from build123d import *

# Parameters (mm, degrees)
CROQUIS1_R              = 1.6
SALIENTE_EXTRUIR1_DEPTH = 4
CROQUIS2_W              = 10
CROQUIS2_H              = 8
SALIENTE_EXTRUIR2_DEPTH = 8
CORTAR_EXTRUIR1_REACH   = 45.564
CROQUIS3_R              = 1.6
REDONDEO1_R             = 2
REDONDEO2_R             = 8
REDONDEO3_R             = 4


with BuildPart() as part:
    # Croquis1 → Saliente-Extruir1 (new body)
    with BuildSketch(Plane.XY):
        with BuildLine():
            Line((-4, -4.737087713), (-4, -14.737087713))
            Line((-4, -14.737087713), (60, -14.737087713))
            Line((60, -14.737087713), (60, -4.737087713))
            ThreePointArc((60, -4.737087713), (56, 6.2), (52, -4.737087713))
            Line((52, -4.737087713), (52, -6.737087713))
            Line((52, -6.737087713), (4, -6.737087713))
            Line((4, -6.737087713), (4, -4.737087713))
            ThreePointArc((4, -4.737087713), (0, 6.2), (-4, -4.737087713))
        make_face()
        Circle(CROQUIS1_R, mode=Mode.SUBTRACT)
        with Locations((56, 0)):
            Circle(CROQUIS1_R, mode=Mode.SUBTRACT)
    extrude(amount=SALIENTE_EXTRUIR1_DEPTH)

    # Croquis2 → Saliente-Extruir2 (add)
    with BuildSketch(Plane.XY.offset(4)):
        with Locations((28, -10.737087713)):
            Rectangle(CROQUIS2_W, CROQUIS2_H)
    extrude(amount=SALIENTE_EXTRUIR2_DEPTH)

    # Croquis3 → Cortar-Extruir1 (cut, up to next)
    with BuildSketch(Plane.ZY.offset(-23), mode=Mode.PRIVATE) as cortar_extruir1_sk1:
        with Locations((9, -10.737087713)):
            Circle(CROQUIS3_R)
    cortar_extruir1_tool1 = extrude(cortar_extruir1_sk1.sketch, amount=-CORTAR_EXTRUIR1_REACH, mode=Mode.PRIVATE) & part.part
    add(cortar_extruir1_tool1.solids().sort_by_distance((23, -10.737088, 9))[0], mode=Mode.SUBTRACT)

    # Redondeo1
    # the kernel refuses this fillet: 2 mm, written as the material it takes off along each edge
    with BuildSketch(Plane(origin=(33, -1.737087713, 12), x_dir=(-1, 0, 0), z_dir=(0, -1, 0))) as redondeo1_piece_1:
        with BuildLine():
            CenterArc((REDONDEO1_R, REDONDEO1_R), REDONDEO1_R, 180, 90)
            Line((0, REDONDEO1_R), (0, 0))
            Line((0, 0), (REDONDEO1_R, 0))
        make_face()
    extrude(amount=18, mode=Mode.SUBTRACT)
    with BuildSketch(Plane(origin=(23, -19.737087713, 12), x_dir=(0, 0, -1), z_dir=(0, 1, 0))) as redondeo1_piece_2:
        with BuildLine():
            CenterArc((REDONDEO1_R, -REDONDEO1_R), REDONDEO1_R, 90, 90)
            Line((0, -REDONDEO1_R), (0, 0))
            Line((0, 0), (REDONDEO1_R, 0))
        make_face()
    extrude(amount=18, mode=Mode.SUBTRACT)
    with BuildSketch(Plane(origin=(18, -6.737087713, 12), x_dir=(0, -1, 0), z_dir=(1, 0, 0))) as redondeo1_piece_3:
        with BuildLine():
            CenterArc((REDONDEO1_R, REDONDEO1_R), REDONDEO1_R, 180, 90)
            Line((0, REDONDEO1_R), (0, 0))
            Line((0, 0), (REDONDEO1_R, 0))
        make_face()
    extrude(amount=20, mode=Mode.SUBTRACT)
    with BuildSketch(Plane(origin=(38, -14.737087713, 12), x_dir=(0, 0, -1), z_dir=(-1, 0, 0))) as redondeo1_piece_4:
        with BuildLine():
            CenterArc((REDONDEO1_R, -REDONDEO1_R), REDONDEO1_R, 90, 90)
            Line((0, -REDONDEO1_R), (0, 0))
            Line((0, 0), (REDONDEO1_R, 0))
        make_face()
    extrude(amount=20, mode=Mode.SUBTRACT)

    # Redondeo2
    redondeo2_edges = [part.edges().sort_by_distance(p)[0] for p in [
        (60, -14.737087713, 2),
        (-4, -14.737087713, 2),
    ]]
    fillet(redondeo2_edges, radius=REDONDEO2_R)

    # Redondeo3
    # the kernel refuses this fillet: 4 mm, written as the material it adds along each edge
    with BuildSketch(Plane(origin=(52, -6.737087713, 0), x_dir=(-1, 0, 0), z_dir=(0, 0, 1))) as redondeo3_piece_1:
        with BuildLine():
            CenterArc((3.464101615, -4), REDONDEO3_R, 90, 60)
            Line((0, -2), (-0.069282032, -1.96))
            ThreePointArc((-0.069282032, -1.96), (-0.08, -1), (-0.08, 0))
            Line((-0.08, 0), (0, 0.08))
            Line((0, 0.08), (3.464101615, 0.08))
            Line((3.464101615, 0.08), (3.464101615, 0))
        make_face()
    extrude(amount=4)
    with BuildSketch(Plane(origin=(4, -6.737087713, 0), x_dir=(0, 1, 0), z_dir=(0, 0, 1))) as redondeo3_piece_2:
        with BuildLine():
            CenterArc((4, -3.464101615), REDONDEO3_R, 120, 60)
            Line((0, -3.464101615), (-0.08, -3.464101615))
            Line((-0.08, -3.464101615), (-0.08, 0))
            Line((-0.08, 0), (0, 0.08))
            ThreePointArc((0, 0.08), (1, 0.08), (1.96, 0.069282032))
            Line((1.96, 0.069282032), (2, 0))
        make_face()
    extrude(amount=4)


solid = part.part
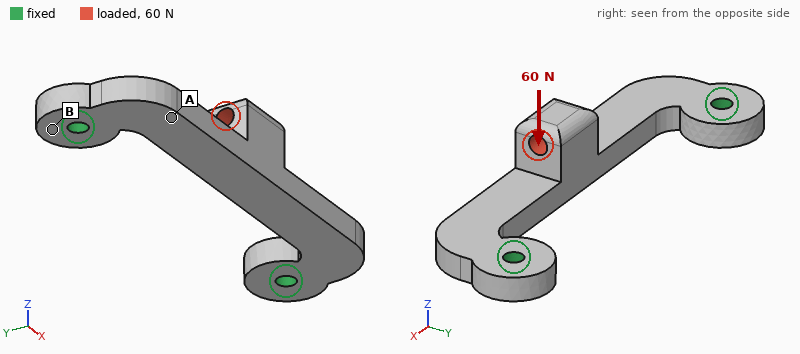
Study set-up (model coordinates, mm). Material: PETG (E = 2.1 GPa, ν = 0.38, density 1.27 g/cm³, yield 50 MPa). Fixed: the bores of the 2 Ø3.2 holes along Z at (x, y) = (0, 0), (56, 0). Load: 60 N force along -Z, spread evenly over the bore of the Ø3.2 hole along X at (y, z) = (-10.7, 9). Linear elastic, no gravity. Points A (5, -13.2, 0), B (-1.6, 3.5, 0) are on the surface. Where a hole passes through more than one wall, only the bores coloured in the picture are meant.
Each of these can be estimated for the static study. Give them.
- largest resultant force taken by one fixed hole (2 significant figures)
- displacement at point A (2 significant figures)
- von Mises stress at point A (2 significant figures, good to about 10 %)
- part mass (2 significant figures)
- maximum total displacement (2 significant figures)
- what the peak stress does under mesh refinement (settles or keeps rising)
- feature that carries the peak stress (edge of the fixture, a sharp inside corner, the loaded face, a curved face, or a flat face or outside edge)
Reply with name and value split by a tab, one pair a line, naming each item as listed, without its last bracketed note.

largest resultant force taken by one fixed hole	30 N
displacement at point A	0.27 mm
von Mises stress at point A	5.4 MPa
part mass	4.4 g
maximum total displacement	0.83 mm
what the peak stress does under mesh refinement	keeps rising
feature that carries the peak stress	edge of the fixture
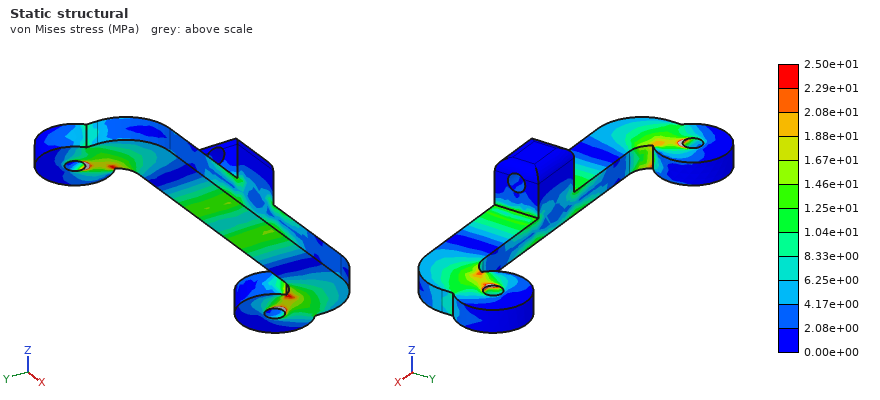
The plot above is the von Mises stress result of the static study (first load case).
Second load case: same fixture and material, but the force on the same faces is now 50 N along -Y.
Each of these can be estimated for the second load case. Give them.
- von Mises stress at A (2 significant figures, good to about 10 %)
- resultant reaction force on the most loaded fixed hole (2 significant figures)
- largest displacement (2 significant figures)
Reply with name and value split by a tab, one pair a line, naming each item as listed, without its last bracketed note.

von Mises stress at A	5.4 MPa
resultant reaction force on the most loaded fixed hole	40 N
largest displacement	0.76 mm
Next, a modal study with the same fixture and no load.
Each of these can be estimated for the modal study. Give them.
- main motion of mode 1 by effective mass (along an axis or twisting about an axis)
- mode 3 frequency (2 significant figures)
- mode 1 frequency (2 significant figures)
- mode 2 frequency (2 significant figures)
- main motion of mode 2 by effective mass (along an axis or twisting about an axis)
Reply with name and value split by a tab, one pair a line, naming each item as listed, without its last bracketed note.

main motion of mode 1 by effective mass	along Z
mode 3 frequency	2600 Hz
mode 1 frequency	1000 Hz
mode 2 frequency	1800 Hz
main motion of mode 2 by effective mass	along Y
